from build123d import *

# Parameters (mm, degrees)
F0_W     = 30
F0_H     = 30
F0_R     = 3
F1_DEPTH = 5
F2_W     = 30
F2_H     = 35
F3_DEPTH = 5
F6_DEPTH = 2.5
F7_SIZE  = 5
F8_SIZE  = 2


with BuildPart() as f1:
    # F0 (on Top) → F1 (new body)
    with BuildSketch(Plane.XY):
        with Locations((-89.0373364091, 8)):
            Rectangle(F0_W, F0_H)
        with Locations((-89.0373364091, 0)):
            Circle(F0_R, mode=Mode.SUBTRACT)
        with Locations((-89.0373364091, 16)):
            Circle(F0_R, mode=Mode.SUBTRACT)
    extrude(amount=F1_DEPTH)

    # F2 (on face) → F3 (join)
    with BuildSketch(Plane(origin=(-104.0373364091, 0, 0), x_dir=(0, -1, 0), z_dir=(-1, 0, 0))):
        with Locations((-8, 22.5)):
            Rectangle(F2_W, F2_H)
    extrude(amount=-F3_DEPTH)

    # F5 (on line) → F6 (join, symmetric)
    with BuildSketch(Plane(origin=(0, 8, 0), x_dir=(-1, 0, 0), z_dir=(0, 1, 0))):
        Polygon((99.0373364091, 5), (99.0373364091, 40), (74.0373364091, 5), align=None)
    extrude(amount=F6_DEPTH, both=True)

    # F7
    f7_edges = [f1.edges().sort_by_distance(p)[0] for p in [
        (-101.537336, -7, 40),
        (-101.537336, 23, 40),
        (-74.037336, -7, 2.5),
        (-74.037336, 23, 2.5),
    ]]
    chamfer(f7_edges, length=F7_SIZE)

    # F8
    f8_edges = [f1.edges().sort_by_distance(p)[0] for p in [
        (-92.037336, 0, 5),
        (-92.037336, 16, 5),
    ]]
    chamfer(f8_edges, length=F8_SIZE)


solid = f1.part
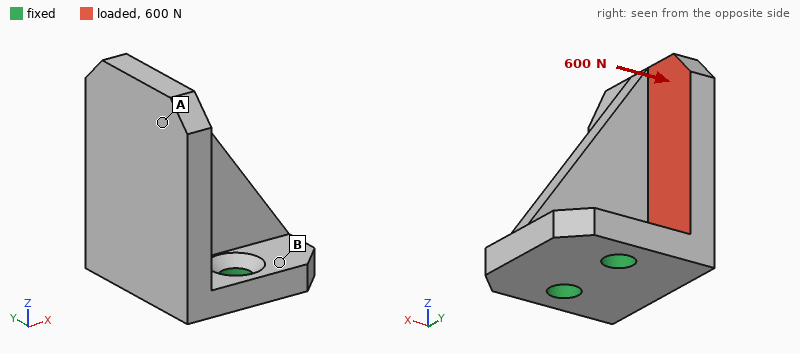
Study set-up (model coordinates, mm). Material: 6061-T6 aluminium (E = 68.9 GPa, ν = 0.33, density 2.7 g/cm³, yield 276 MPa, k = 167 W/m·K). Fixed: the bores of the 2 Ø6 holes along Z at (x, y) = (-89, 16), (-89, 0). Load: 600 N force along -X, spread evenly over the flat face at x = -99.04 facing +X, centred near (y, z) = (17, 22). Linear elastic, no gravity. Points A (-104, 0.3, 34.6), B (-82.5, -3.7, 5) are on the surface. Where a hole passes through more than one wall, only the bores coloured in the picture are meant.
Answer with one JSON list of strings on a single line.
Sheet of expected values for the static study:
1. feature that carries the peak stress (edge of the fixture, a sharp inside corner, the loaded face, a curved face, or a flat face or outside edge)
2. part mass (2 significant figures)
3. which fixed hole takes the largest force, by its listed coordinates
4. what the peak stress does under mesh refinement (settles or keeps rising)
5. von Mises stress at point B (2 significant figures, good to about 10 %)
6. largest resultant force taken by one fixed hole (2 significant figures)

["edge of the fixture", "31 g", "(-89, 16)", "keeps rising", "21 MPa", "560 N"]
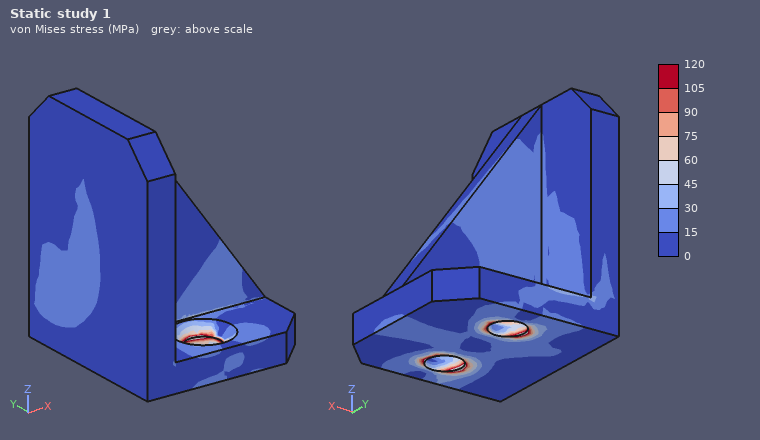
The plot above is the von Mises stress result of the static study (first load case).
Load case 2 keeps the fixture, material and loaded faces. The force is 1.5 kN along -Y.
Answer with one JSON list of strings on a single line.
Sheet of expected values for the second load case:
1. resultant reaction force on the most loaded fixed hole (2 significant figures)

["2.1 kN"]
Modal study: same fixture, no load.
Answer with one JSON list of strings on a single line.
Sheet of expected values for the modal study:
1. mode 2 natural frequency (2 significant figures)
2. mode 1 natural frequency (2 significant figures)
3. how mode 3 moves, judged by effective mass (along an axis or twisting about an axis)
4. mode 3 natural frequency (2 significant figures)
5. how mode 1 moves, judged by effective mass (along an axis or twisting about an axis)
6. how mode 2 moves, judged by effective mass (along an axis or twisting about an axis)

["4900 Hz", "3800 Hz", "twisting about Z", "9600 Hz", "along X", "along Y"]
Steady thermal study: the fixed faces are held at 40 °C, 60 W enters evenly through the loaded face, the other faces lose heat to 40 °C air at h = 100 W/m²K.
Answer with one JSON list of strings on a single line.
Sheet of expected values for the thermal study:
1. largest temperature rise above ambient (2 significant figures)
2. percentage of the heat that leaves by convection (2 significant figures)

["50 K", "16 %"]
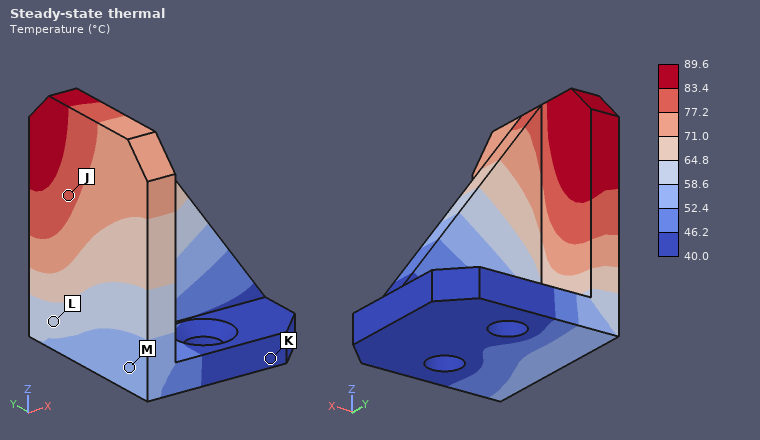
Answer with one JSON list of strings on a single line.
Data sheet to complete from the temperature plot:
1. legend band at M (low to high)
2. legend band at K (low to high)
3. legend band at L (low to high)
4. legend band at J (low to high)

["52.4 to 58.6 °C", "40.0 to 46.2 °C", "58.6 to 64.8 °C", "77.2 to 83.4 °C"]
